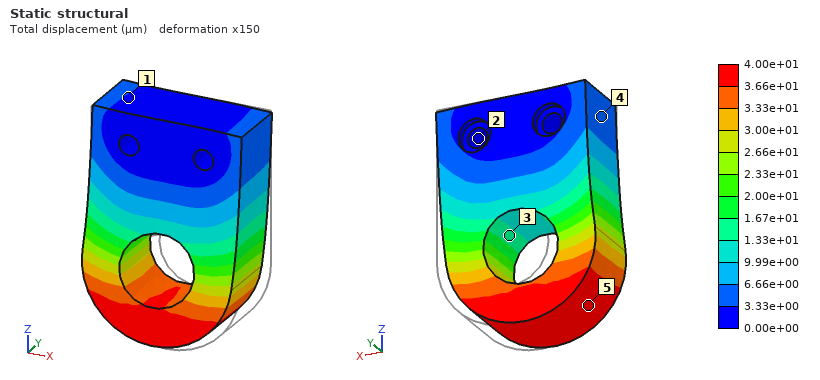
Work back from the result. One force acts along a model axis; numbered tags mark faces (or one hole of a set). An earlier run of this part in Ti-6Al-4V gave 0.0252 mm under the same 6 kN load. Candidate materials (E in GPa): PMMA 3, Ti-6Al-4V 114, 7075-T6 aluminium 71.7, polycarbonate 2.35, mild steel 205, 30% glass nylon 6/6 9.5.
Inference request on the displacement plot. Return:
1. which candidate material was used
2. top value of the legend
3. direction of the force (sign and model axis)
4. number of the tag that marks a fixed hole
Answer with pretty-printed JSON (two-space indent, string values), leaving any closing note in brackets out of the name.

{
  "which candidate material was used": "7075-T6 aluminium",
  "top value of the legend": "4.00e+01 µm",
  "direction of the force": "-X",
  "number of the tag that marks a fixed hole": "2"
}
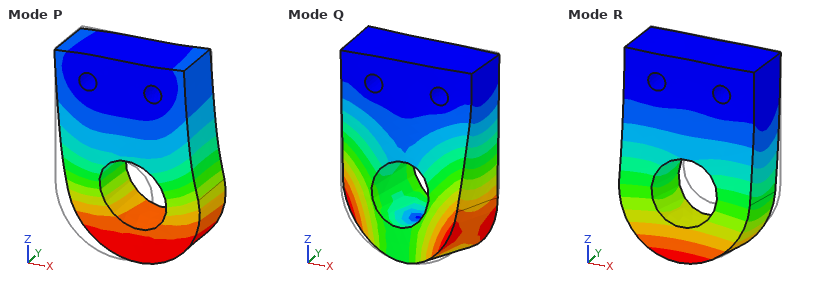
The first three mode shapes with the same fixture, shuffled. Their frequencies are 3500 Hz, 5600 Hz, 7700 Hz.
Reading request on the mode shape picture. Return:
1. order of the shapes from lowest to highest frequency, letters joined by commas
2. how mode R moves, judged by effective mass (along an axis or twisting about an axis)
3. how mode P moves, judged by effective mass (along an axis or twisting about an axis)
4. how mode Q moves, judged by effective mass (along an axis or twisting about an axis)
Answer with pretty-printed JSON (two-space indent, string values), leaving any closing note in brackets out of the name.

{
  "order of the shapes from lowest to highest frequency, letters joined by commas": "R, P, Q",
  "how mode R moves, judged by effective mass": "along Y",
  "how mode P moves, judged by effective mass": "along X",
  "how mode Q moves, judged by effective mass": "twisting about Z"
}
